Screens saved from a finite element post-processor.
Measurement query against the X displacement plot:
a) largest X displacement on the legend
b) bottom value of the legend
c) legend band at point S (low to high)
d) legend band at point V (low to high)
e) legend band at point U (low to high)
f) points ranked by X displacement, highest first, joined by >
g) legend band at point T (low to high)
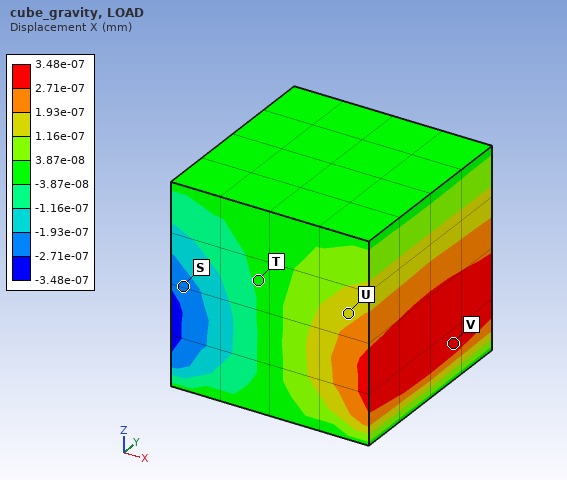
3.48e-07 mm
-3.48e-07 mm
-2.71e-07 to -1.93e-07 mm
2.71e-07 to 3.48e-07 mm
1.16e-07 to 1.93e-07 mm
V > U > T > S
-3.87e-08 to 3.87e-08 mm
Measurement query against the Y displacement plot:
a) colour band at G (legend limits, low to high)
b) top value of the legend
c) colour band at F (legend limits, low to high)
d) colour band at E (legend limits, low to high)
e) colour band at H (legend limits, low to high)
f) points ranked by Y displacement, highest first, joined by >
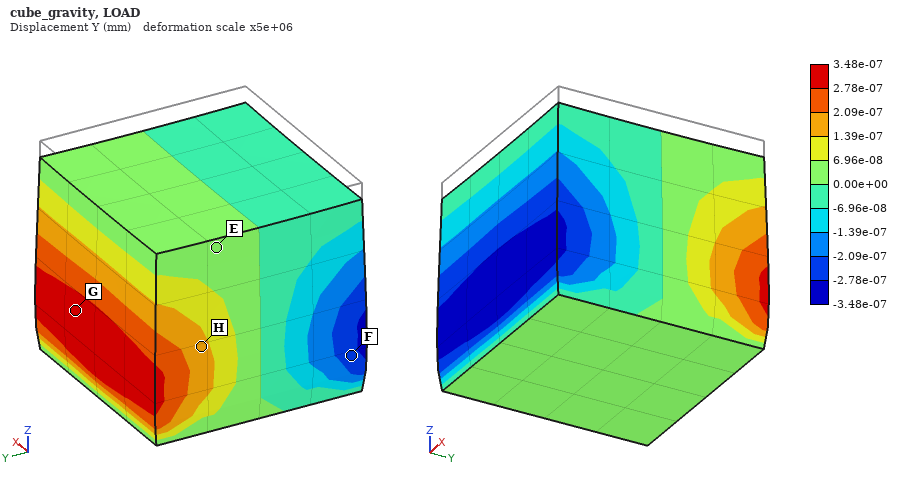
2.78e-07 to 3.48e-07 mm
3.48e-07 mm
-2.78e-07 to -2.09e-07 mm
0.00e+00 to 6.96e-08 mm
1.39e-07 to 2.09e-07 mm
G > H > E > F
